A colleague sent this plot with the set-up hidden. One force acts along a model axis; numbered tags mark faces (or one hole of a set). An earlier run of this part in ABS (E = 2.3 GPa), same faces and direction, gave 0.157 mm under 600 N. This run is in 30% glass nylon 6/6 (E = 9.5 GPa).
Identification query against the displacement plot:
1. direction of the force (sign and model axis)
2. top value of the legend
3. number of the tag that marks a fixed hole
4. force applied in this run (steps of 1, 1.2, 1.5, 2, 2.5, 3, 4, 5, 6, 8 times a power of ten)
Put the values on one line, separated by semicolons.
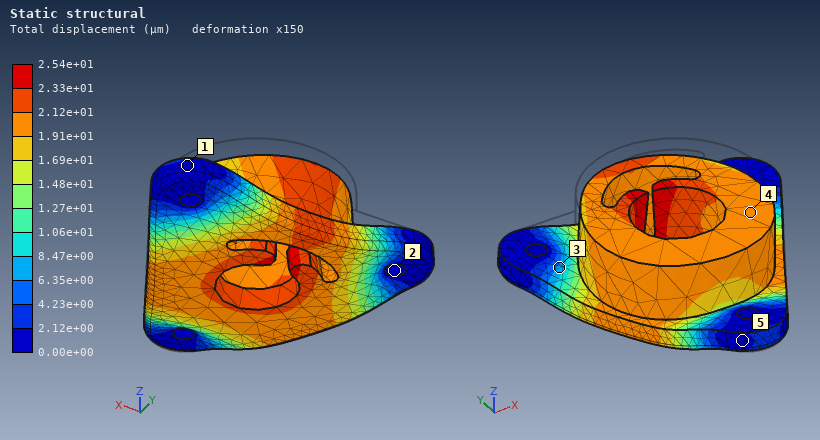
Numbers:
-Z; 2.54e+01 µm; 2; 400 N
